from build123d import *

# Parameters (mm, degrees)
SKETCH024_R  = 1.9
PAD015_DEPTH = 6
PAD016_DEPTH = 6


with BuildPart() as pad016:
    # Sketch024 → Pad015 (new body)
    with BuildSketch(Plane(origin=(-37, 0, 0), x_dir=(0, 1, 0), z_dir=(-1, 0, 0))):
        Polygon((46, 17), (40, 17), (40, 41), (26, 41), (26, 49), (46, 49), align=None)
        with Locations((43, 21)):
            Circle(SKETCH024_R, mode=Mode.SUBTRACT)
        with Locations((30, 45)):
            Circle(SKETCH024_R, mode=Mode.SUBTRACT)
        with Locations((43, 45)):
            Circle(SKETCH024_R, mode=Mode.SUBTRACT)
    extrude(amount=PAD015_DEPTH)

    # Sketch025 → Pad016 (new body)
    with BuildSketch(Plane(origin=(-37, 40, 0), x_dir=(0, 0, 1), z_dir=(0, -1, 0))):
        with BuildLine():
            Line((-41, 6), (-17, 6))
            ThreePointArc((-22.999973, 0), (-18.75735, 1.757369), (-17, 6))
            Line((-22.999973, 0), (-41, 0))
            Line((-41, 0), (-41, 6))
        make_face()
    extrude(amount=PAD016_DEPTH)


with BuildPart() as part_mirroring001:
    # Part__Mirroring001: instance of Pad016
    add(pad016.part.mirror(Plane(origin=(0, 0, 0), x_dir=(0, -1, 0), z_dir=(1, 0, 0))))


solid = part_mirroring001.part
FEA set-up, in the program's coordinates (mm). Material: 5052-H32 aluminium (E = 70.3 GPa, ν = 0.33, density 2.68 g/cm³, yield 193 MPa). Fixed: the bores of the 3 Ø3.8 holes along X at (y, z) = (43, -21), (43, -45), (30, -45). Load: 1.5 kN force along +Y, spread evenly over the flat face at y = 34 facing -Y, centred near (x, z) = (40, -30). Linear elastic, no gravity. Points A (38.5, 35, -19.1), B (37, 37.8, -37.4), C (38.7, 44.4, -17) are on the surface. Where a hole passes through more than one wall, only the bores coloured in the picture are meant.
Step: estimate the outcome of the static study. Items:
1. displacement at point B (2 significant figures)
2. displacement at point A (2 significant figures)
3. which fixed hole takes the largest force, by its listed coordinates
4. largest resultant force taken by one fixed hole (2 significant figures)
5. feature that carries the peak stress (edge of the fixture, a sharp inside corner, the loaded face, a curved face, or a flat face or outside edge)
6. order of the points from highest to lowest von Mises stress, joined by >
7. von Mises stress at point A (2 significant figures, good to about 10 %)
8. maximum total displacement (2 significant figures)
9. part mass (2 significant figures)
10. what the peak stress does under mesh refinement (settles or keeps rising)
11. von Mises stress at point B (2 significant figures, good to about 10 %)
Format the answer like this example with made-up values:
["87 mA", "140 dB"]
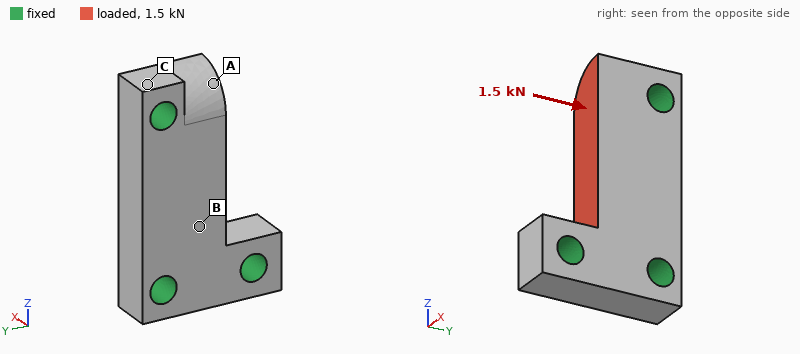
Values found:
["2.5 µm", "1.2 µm", "(43, -21)", "910 N", "edge of the fixture", "B > A > C", "11 MPa", "3.9 µm", "6.5 g", "keeps rising", "15 MPa"]
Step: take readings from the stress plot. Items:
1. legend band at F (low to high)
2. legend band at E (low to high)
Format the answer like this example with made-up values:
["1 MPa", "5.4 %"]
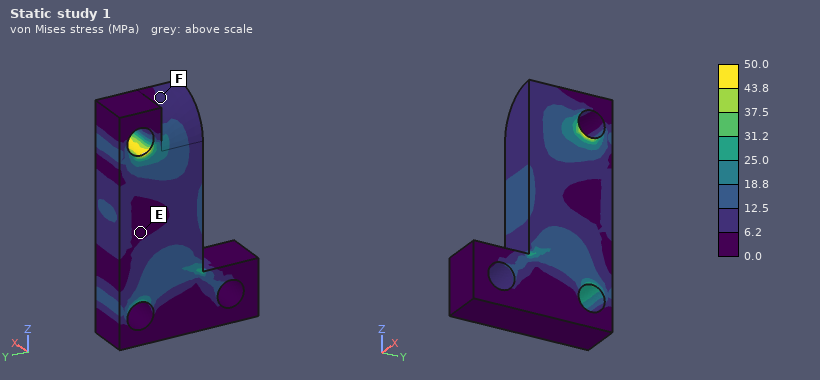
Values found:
["6.2 to 12.5 MPa", "0.0 to 6.2 MPa"]
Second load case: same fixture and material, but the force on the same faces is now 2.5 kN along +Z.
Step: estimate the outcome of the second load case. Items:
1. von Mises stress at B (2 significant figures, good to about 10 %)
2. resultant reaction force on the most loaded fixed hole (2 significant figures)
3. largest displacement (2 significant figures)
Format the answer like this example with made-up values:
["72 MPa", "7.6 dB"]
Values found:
["26 MPa", "1.3 kN", "12 µm"]
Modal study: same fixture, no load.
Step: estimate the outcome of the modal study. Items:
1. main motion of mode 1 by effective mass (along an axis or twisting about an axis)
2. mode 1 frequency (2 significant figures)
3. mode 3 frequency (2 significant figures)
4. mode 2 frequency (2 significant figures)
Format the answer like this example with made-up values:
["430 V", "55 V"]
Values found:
["along X", "38 kHz", "54 kHz", "53 kHz"]
